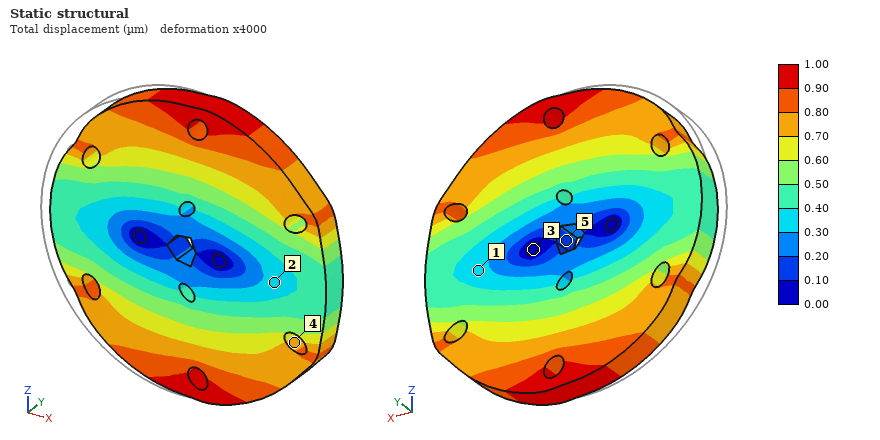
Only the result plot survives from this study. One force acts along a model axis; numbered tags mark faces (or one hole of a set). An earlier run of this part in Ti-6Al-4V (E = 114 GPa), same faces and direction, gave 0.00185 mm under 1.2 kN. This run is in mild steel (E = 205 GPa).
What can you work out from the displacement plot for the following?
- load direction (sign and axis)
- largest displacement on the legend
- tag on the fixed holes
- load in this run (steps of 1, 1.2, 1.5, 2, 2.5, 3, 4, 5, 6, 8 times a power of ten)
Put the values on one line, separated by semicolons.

+X; 1.00 µm; 3; 1.2 kN
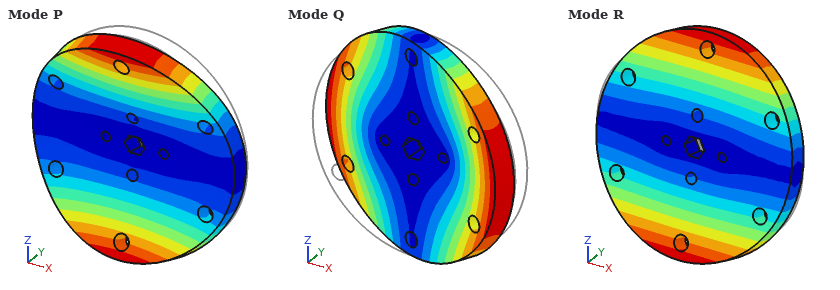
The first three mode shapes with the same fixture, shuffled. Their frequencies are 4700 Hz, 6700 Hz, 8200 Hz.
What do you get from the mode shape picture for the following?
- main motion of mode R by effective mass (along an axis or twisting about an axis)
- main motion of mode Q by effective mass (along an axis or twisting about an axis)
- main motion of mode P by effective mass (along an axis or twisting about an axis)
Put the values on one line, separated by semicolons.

twisting about X; twisting about Z; along Y
